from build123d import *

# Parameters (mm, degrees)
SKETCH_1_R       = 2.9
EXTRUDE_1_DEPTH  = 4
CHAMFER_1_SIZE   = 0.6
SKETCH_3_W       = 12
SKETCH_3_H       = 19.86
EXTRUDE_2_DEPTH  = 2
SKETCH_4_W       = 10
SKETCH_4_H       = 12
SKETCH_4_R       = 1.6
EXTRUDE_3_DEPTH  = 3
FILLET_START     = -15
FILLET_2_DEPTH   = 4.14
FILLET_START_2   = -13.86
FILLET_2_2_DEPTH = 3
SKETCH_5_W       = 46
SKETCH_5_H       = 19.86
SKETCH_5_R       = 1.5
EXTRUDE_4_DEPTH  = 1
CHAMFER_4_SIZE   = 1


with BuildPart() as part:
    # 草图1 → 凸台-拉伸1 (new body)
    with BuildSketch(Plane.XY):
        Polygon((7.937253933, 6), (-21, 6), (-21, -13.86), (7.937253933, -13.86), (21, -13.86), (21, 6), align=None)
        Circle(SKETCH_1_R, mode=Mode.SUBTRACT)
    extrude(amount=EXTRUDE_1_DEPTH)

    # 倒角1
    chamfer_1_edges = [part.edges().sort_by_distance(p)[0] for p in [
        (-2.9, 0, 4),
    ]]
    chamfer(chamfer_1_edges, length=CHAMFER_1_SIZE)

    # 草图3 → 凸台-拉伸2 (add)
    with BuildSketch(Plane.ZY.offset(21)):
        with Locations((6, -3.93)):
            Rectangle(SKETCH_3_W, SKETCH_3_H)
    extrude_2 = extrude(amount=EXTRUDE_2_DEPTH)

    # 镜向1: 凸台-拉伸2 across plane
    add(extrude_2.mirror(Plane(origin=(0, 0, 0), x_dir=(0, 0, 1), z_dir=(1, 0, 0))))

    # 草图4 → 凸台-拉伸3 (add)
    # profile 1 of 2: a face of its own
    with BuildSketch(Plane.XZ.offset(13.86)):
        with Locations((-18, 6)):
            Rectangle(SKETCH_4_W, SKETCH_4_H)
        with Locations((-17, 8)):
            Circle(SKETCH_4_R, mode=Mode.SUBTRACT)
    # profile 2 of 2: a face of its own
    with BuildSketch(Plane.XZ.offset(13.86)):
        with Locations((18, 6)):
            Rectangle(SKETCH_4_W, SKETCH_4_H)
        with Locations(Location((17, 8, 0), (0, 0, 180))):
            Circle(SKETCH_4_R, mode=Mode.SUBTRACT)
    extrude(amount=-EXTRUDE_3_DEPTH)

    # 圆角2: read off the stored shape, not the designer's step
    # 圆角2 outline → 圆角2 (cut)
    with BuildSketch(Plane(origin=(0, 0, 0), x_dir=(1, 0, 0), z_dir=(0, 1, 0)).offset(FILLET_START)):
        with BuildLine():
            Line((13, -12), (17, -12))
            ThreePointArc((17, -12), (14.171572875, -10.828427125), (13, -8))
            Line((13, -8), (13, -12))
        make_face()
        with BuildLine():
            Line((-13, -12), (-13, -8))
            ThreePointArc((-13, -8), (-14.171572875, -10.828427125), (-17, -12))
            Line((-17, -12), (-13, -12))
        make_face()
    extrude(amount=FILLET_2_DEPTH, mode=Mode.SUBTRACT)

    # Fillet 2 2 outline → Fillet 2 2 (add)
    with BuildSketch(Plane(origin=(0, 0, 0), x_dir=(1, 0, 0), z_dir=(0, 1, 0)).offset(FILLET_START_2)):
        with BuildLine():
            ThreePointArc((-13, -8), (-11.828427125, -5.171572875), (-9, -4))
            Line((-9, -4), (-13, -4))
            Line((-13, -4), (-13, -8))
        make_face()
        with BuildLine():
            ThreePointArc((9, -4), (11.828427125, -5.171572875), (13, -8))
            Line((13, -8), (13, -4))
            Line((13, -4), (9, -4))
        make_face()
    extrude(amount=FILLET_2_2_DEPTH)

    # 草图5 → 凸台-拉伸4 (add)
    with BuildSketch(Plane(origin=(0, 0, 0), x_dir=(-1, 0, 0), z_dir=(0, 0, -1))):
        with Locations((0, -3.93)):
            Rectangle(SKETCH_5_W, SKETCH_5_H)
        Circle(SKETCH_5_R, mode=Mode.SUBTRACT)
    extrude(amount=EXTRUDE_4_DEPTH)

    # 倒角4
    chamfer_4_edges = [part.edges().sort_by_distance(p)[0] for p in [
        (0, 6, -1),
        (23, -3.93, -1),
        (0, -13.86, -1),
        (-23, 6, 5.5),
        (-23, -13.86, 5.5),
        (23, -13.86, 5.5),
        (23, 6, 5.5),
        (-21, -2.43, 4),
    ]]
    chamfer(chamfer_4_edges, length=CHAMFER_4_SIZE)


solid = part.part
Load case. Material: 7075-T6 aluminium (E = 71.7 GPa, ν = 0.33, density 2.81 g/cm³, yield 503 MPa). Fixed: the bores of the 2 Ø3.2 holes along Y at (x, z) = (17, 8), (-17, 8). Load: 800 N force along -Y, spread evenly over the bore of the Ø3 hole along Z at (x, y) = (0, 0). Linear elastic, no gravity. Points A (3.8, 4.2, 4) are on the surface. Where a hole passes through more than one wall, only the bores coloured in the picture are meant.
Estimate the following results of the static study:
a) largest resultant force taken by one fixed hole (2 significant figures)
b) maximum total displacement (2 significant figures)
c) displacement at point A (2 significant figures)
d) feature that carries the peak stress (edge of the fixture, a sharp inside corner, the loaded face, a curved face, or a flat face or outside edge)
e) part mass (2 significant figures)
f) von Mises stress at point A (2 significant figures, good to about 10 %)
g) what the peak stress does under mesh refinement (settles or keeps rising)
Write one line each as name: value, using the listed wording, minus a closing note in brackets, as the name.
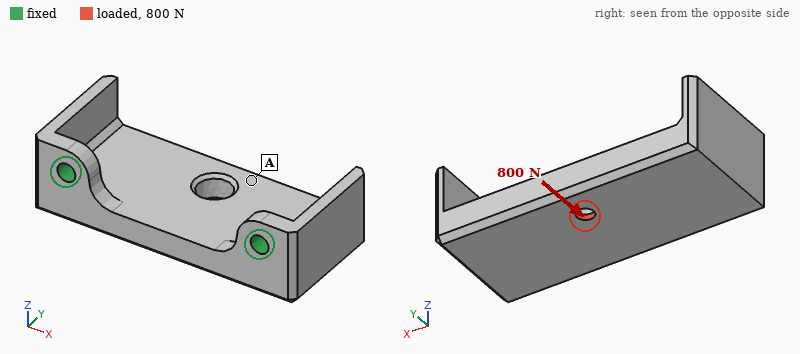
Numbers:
largest resultant force taken by one fixed hole: 410 N
maximum total displacement: 84 µm
displacement at point A: 70 µm
feature that carries the peak stress: edge of the fixture
part mass: 15 g
von Mises stress at point A: 27 MPa
what the peak stress does under mesh refinement: keeps rising
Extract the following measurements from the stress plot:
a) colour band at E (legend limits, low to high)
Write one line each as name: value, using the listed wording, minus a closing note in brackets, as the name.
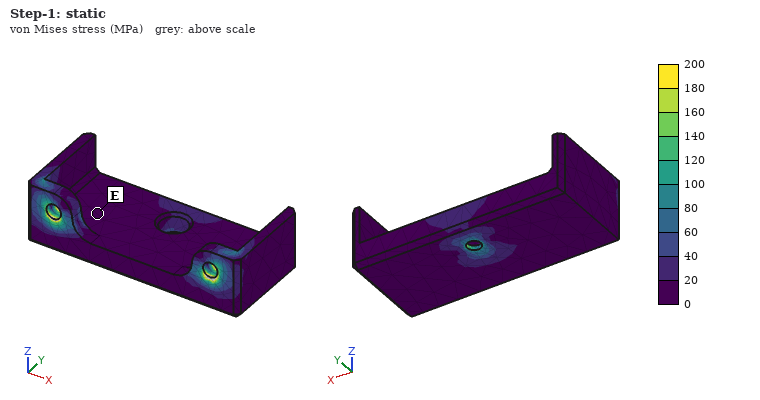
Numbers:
colour band at E: 0 to 20 MPa
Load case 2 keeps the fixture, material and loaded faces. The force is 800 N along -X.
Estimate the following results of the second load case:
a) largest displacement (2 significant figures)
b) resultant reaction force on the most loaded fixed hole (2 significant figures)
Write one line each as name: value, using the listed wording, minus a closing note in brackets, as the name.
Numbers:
largest displacement: 13 µm
resultant reaction force on the most loaded fixed hole: 500 N
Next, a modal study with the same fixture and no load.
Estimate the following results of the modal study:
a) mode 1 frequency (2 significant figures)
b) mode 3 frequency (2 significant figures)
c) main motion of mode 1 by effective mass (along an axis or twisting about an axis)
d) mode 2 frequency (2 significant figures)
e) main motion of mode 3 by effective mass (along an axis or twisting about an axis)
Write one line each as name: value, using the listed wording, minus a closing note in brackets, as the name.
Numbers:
mode 1 frequency: 4500 Hz
mode 3 frequency: 15 kHz
main motion of mode 1 by effective mass: along Z
mode 2 frequency: 8600 Hz
main motion of mode 3 by effective mass: along X
